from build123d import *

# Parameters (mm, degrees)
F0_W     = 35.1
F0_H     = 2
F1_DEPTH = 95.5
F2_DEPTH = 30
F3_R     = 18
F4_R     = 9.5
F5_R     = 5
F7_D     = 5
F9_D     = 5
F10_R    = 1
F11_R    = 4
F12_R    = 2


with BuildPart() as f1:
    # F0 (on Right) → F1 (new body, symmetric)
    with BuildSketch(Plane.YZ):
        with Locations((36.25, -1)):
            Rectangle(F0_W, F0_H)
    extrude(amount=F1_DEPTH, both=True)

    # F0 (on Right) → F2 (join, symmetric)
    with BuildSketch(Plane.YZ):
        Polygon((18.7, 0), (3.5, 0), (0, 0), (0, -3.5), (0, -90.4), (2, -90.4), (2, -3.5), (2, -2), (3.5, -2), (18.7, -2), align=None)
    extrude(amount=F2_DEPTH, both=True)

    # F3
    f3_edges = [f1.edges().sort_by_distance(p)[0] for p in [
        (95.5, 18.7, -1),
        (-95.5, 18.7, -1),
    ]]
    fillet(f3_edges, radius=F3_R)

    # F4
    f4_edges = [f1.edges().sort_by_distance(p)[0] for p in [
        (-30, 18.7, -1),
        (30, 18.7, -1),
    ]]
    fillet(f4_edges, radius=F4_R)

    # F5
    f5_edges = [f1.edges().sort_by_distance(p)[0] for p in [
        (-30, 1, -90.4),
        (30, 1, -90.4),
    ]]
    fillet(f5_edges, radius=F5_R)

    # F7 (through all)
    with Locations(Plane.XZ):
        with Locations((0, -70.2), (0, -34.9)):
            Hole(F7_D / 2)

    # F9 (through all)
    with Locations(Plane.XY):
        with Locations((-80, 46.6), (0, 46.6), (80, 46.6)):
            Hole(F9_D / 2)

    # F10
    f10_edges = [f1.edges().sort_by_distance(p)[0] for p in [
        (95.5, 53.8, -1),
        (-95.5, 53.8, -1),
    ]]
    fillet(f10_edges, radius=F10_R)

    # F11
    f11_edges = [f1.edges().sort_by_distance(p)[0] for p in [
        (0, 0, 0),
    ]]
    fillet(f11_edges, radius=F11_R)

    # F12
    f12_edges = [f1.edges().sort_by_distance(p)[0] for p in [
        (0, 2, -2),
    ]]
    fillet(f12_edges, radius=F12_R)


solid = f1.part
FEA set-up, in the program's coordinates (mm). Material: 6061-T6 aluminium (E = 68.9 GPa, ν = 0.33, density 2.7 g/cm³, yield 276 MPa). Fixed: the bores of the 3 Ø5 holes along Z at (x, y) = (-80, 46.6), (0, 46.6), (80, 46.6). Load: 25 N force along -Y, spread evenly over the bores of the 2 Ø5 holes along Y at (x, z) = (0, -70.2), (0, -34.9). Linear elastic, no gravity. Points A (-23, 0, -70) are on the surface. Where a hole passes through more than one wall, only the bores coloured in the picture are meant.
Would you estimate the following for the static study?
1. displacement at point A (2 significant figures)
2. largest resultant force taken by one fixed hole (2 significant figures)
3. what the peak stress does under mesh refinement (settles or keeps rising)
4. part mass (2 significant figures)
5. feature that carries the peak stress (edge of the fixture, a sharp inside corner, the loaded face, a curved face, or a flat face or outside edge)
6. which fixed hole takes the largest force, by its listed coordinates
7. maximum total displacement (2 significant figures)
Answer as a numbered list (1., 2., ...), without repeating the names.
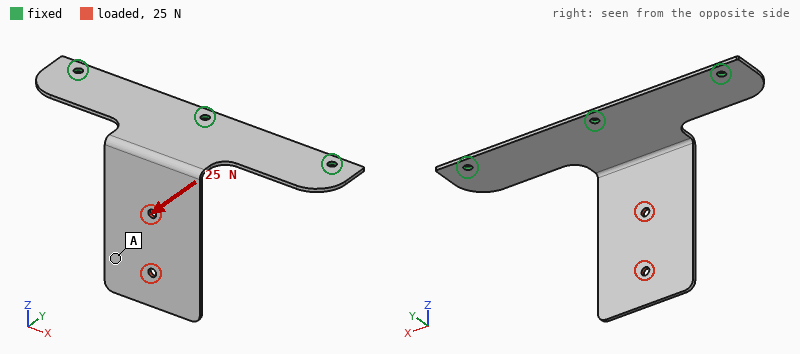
1. 1.8 mm
2. 22 N
3. keeps rising
4. 69 g
5. edge of the fixture
6. (0, 46.6)
7. 2.4 mm
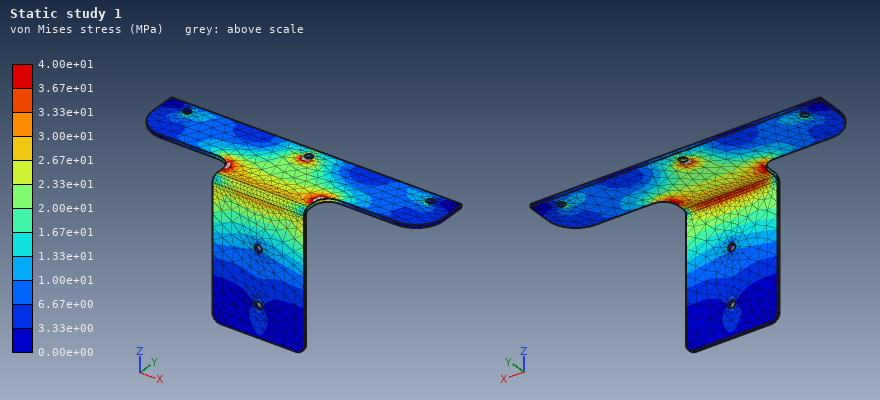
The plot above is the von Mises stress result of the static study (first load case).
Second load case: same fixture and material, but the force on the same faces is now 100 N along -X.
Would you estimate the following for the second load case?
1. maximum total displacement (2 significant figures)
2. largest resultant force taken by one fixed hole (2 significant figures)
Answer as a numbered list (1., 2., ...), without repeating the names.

1. 2.5 mm
2. 59 N
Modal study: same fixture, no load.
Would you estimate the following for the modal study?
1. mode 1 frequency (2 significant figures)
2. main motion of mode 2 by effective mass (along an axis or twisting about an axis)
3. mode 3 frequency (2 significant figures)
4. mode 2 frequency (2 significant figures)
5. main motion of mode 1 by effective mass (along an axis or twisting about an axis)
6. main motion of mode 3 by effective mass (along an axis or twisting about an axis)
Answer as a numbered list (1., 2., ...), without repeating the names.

1. 120 Hz
2. along X
3. 390 Hz
4. 230 Hz
5. along Y
6. along Z
